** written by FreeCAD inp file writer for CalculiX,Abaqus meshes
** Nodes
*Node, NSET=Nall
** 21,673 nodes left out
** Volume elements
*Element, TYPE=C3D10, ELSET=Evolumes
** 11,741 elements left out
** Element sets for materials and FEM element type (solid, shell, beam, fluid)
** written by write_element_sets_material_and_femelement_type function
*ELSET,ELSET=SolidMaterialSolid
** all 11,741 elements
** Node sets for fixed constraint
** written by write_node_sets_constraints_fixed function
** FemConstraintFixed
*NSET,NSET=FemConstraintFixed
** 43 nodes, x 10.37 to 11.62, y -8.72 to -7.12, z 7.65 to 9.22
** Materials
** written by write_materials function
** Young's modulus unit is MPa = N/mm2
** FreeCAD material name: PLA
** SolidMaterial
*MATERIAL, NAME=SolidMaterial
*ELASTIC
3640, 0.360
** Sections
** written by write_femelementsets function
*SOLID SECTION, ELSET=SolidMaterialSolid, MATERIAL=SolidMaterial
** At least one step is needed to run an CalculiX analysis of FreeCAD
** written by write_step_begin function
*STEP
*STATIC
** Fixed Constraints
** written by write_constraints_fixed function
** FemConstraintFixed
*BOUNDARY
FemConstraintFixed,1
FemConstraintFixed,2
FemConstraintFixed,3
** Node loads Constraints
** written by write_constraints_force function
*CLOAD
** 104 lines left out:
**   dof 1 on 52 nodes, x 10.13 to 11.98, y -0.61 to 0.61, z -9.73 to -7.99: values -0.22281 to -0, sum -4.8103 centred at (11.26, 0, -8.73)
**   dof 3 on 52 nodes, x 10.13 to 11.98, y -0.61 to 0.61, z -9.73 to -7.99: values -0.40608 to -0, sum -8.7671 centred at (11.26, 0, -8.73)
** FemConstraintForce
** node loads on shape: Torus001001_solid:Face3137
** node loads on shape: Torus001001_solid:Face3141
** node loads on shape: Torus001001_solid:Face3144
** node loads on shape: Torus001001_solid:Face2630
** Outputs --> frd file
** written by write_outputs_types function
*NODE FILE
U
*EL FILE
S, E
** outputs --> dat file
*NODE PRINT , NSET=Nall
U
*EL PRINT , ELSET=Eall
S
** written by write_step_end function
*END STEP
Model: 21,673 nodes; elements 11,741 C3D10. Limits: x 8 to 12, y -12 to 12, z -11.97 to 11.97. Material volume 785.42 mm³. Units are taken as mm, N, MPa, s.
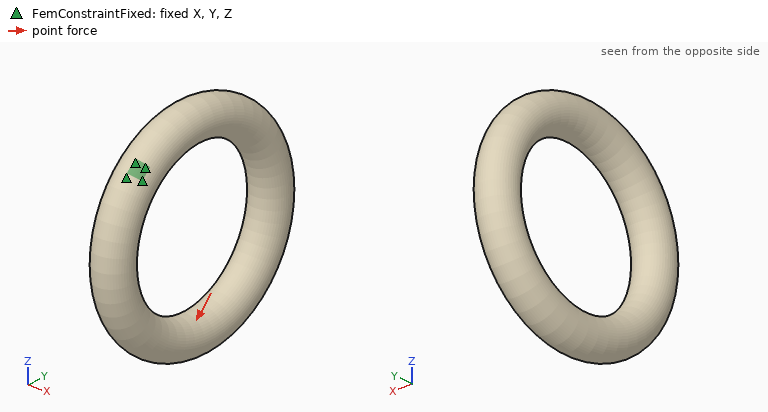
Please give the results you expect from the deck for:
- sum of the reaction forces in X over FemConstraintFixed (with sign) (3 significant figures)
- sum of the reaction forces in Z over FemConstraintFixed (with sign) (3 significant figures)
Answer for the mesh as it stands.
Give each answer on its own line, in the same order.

4.81 N
8.77 N
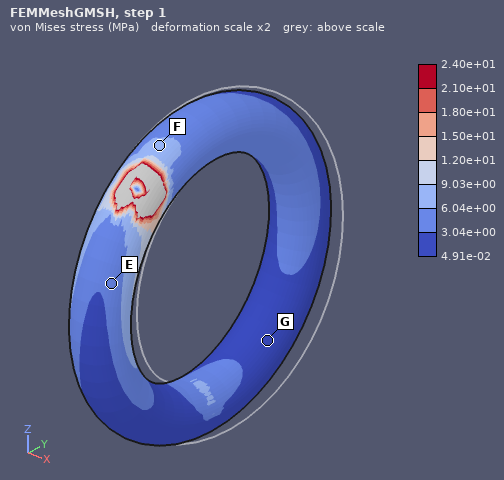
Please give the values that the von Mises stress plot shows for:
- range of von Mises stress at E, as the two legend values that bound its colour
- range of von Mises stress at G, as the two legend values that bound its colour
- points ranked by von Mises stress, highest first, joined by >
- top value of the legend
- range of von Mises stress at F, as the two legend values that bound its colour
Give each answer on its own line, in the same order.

3.04e+00 to 6.04e+00 MPa
4.91e-02 to 3.04e+00 MPa
F > E > G
2.40e+01 MPa
6.04e+00 to 9.03e+00 MPa
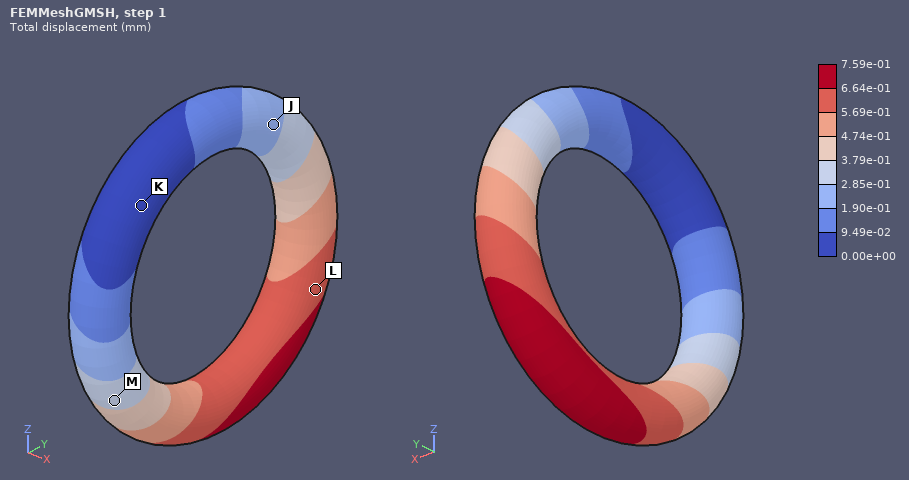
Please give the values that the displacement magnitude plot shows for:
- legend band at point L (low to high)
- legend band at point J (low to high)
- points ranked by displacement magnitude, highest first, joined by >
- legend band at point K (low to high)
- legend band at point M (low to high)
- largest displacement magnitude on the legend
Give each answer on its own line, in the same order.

5.69e-01 to 6.64e-01 mm
1.90e-01 to 2.85e-01 mm
L > M > J > K
0.00e+00 to 9.49e-02 mm
2.85e-01 to 3.79e-01 mm
7.59e-01 mm
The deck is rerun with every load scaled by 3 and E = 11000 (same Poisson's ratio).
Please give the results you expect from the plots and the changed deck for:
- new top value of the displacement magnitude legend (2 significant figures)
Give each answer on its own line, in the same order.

0.75 mm
